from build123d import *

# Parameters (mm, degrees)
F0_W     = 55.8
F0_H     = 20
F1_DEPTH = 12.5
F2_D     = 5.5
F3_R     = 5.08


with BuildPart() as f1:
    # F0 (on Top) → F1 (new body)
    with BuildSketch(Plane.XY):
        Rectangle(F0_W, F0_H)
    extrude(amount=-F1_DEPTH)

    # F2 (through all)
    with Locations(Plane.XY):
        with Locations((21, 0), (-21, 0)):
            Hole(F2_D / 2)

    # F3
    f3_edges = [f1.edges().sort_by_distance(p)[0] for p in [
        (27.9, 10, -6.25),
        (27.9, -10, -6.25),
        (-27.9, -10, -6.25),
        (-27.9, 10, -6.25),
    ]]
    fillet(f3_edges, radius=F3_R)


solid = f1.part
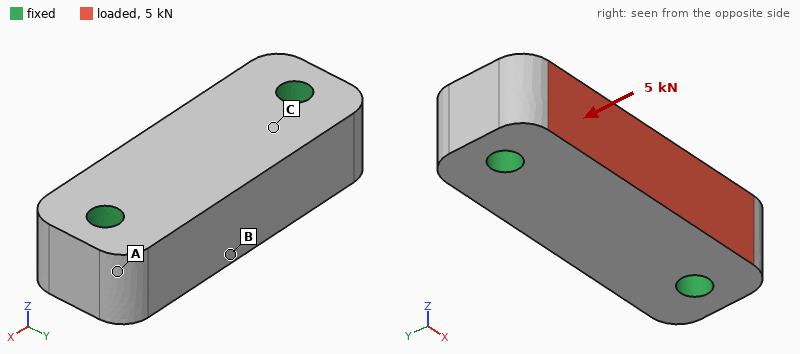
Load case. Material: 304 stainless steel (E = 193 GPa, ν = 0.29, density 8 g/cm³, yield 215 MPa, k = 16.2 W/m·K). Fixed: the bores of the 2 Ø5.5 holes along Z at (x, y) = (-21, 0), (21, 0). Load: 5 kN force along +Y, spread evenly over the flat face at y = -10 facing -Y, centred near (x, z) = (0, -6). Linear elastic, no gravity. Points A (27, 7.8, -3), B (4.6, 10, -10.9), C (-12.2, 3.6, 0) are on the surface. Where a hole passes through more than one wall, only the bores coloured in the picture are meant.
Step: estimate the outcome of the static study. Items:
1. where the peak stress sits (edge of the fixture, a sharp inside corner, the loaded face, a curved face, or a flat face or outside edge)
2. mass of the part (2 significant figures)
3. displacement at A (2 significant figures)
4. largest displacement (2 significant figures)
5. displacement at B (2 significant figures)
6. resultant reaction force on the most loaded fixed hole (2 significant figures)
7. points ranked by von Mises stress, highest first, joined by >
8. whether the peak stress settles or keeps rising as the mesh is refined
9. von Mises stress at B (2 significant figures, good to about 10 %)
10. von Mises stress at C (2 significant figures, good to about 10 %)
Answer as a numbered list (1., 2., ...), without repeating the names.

1. edge of the fixture
2. 100 g
3. 0.67 µm
4. 2.8 µm
5. 2.3 µm
6. 2.5 kN
7. B > C > A
8. keeps rising
9. 17 MPa
10. 13 MPa
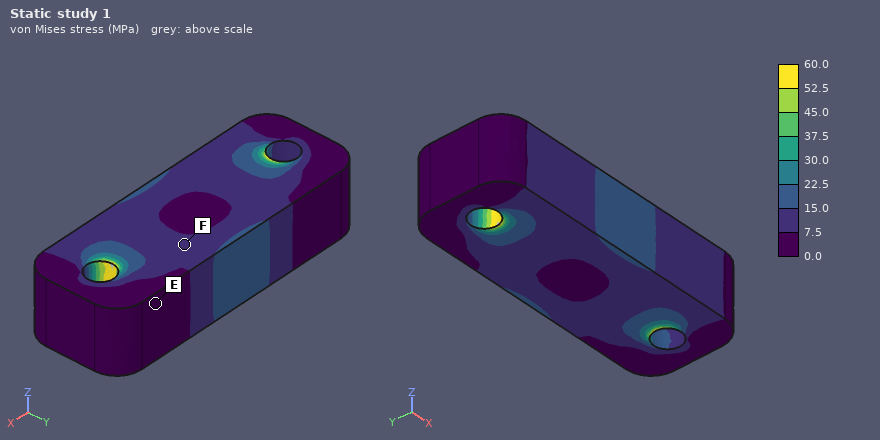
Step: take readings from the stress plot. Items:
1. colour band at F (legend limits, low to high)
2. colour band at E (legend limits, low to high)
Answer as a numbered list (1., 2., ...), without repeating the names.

1. 7.5 to 15.0 MPa
2. 0.0 to 7.5 MPa
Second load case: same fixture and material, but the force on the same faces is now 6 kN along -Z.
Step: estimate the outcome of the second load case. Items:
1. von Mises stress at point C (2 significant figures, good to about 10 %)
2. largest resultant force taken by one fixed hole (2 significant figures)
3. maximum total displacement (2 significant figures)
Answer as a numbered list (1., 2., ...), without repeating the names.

1. 29 MPa
2. 3.0 kN
3. 11 µm
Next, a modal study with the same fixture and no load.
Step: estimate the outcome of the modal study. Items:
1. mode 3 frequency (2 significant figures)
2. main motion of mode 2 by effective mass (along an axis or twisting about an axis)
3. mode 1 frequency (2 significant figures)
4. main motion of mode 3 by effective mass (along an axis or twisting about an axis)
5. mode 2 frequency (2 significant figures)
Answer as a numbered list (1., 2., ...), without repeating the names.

1. 30 kHz
2. along Y
3. 24 kHz
4. twisting about X
5. 25 kHz
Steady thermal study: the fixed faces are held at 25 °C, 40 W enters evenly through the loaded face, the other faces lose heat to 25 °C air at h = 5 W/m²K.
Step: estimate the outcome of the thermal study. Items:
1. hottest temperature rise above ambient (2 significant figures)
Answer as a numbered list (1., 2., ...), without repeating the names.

1. 78 K
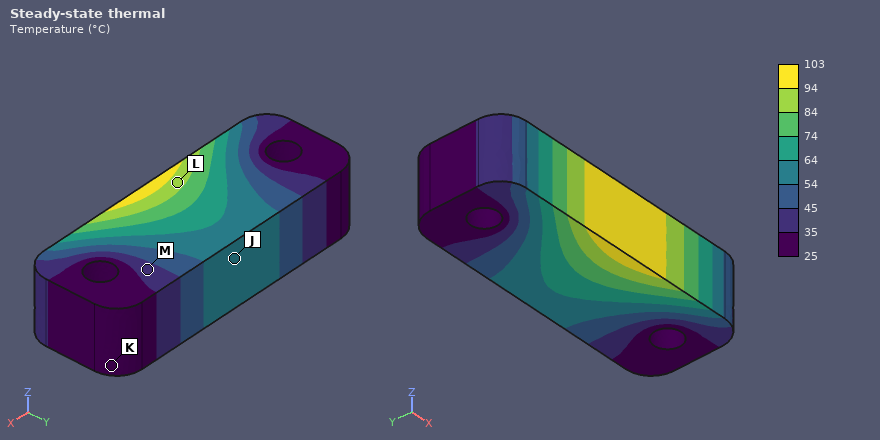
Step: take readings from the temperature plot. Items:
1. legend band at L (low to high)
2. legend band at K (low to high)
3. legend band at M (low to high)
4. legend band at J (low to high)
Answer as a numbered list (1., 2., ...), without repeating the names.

1. 84 to 94 °C
2. 25 to 35 °C
3. 35 to 45 °C
4. 54 to 64 °C
